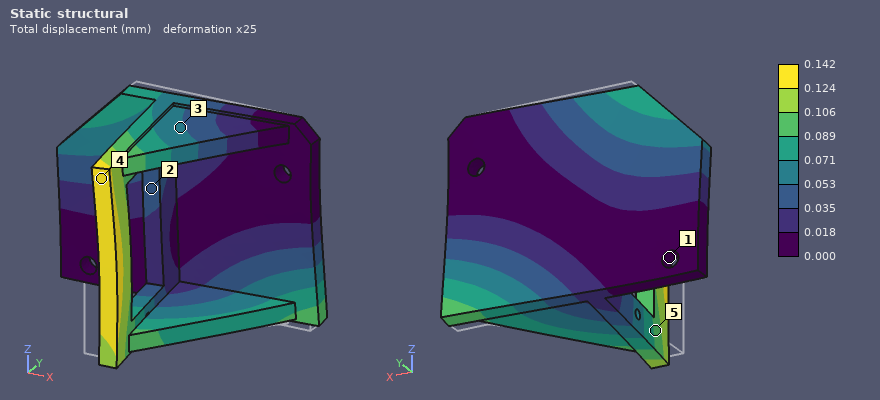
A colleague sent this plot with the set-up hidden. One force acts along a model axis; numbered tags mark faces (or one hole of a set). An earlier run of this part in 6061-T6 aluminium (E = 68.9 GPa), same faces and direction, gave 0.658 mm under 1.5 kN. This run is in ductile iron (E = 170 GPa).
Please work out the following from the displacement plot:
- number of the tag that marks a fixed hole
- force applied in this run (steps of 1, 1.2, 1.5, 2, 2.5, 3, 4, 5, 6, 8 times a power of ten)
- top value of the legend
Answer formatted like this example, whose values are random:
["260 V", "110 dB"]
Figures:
["1", "800 N", "0.142 mm"]
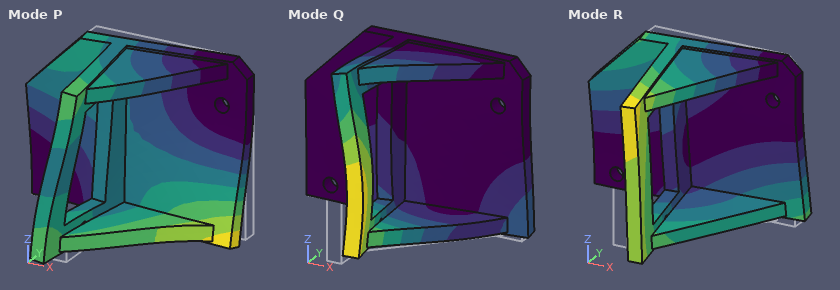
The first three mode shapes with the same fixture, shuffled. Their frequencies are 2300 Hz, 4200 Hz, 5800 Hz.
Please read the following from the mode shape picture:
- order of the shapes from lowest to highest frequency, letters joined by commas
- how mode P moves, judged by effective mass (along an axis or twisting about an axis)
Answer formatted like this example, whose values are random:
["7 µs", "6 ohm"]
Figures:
["R, P, Q", "along Y"]
